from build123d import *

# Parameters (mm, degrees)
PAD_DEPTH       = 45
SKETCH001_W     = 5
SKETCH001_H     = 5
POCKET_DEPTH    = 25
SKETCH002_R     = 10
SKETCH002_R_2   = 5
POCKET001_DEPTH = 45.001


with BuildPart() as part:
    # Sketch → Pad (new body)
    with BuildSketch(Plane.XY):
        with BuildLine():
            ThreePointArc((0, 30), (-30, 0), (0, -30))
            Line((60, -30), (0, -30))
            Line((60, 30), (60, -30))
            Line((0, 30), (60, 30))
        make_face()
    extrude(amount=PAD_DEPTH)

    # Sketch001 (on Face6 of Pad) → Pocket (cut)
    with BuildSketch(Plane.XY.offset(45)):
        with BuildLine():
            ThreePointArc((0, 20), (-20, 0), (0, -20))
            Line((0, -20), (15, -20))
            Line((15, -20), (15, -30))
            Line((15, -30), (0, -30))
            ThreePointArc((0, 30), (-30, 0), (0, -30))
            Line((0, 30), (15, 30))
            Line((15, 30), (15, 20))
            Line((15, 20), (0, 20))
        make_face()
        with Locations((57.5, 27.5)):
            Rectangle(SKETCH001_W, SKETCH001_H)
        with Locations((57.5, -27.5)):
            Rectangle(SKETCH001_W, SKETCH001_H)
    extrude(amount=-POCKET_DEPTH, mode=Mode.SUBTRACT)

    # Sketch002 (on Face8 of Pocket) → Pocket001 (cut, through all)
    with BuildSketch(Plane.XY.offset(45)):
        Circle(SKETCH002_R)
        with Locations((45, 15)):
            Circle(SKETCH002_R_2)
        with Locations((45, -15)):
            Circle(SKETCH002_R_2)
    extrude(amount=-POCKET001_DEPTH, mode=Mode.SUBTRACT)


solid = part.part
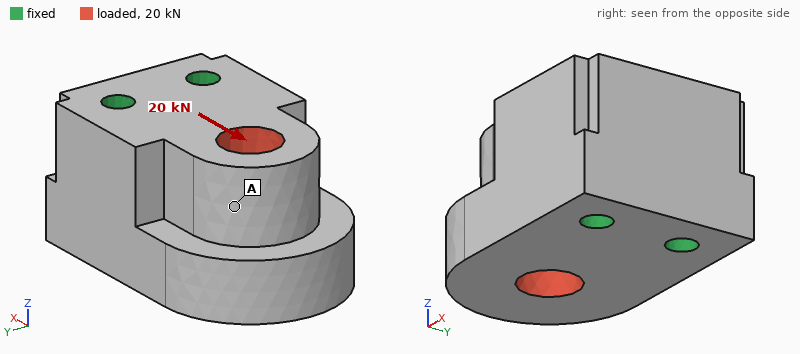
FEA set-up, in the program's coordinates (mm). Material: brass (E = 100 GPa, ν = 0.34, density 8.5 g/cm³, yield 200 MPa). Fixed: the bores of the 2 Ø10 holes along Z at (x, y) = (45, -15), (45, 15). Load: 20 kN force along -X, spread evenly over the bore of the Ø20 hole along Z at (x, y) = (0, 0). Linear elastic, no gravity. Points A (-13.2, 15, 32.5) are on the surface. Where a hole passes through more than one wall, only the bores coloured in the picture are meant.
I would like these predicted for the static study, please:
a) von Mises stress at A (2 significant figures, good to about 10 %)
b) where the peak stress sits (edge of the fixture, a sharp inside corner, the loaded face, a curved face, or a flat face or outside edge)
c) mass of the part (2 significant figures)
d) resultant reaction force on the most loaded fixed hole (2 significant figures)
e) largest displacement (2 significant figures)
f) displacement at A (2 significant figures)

5.0 MPa
the loaded face
1.5 kg
10 kN
8.9 µm
5.1 µm
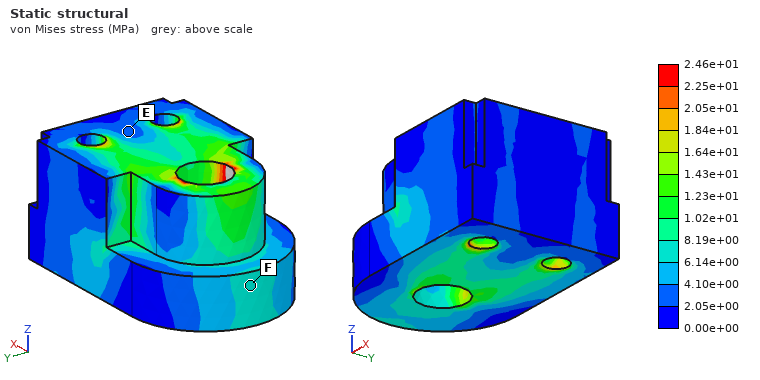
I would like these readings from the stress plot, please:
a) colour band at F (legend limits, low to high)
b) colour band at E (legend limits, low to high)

6.14e+00 to 8.19e+00 MPa
2.05e+00 to 4.10e+00 MPa
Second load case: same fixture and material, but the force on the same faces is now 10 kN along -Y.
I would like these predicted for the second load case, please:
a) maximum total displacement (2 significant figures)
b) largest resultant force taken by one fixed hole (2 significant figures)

19 µm
13 kN
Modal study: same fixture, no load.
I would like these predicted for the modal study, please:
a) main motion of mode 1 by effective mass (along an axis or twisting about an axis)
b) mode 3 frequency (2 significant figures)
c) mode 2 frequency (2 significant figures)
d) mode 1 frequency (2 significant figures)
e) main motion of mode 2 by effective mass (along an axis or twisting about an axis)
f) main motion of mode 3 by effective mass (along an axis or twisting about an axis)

along Z
8100 Hz
5100 Hz
4800 Hz
along Y
twisting about X
